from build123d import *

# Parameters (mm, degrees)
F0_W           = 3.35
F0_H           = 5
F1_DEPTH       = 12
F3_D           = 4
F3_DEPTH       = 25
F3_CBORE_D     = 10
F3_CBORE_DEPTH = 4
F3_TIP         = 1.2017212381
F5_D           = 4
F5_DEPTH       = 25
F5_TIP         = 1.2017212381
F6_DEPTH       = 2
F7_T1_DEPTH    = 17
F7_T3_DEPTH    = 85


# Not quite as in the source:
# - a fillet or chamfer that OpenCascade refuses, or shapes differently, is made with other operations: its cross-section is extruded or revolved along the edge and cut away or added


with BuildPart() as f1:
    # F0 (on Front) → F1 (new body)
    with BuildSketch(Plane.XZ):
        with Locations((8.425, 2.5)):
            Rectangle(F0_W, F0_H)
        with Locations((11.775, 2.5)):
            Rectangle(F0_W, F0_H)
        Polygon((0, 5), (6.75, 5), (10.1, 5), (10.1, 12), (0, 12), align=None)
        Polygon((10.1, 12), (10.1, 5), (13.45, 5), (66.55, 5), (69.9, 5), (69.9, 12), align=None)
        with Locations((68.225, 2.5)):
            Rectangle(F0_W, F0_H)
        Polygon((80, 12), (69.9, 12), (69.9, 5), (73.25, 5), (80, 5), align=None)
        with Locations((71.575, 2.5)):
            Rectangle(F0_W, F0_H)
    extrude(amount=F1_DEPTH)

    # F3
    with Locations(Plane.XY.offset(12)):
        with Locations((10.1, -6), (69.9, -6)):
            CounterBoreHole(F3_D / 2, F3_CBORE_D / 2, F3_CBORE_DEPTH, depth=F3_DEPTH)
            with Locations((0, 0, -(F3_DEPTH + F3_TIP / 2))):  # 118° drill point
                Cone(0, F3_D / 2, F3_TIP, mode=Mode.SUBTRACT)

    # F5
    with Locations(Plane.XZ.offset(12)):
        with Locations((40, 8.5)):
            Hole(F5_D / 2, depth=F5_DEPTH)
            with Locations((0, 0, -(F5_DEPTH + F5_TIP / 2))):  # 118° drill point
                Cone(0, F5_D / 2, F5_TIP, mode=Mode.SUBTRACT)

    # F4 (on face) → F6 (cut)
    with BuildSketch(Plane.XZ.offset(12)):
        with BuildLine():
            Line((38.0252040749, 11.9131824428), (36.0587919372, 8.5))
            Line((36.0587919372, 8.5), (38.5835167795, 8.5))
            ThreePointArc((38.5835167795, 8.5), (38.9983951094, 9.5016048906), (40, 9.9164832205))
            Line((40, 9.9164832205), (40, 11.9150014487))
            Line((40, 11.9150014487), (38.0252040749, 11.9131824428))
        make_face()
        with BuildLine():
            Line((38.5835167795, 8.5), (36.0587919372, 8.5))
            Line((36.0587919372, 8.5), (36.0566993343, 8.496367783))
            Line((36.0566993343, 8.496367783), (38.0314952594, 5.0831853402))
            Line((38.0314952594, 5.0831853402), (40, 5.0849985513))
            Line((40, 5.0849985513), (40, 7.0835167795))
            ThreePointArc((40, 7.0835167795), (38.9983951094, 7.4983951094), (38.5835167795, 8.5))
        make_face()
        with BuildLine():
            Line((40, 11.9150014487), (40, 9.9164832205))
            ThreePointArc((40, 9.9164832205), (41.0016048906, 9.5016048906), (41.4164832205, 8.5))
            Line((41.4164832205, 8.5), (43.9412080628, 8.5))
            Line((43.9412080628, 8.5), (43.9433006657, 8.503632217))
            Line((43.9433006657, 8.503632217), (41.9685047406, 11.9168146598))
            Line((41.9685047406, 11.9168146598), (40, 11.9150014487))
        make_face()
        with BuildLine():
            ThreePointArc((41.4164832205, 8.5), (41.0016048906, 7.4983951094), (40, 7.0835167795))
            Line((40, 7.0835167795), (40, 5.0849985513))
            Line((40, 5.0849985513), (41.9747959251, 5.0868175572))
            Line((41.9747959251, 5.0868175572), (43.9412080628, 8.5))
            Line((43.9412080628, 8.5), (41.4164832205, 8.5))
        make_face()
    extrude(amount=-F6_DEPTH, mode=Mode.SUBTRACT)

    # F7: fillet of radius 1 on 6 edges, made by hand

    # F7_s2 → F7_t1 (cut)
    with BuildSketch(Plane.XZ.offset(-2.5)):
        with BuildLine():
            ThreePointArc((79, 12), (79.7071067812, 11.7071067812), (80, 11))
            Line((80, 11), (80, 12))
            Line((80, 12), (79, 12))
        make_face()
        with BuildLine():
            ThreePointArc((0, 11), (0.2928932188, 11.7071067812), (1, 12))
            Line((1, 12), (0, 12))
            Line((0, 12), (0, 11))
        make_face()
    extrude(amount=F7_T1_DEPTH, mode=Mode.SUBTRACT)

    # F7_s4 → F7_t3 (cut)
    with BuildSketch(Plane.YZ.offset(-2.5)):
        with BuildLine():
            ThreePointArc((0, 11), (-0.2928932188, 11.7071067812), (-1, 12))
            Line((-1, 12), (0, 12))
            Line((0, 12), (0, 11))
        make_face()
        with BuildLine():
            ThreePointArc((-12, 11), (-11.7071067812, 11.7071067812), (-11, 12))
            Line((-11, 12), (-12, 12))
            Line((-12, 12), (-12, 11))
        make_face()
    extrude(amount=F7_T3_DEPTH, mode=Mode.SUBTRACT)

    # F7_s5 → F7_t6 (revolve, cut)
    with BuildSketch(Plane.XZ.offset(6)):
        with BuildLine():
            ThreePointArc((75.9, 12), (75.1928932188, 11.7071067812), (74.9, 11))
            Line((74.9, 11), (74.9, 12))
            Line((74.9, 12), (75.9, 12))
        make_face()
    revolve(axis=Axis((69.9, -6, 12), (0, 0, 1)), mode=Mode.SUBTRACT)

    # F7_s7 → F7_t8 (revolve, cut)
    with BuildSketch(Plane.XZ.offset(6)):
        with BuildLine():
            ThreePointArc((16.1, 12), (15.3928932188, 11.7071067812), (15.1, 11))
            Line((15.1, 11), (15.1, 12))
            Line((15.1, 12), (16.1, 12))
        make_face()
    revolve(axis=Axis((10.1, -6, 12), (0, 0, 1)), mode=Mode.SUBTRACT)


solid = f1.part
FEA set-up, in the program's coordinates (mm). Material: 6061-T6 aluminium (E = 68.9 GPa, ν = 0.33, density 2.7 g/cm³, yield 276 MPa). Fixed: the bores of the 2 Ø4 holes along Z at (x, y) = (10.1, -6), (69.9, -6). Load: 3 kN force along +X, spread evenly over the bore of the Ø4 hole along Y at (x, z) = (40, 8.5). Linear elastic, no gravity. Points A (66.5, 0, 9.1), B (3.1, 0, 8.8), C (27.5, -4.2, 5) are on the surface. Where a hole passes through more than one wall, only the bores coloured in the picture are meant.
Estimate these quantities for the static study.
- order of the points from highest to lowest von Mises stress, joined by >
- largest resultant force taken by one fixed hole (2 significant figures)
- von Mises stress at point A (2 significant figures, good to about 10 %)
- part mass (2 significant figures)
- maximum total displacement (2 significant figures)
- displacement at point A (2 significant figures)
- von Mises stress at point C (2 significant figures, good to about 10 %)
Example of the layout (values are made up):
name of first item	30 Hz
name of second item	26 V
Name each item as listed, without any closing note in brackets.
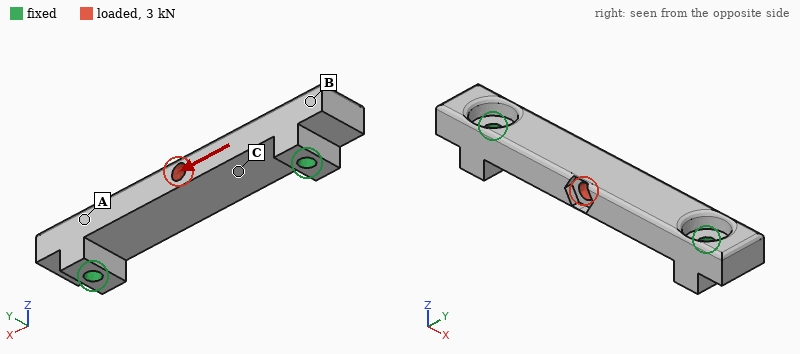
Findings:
order of the points from highest to lowest von Mises stress, joined by >	C > A > B
largest resultant force taken by one fixed hole	1.5 kN
von Mises stress at point A	18 MPa
part mass	17 g
maximum total displacement	12 µm
displacement at point A	4.1 µm
von Mises stress at point C	30 MPa
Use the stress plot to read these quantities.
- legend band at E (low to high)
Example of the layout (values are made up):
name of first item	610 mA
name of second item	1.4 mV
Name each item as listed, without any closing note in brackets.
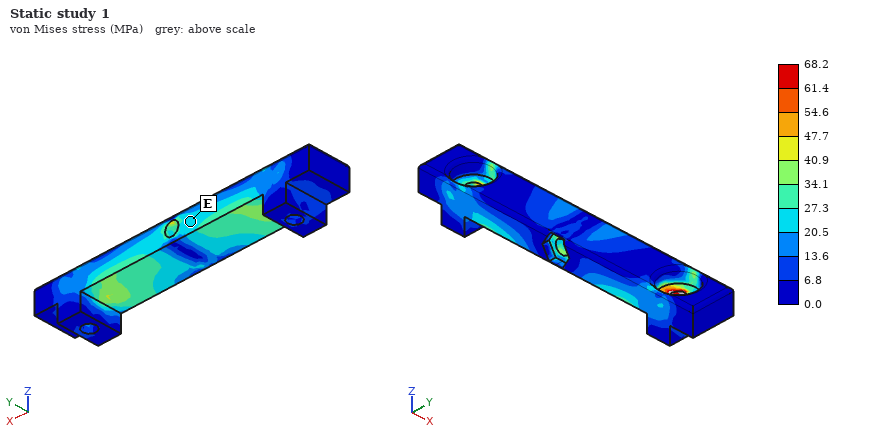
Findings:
legend band at E	20.5 to 27.3 MPa
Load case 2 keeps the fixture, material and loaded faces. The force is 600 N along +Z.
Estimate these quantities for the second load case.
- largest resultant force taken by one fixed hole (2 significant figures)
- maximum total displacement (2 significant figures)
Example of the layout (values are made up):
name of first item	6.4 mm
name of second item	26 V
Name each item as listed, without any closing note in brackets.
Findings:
largest resultant force taken by one fixed hole	540 N
maximum total displacement	48 µm
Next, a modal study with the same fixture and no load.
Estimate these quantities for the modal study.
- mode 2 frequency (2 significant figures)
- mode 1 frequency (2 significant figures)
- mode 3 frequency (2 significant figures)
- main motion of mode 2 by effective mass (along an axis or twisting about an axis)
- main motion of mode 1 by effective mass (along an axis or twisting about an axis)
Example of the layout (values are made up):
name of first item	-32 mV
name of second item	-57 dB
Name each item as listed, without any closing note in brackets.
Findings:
mode 2 frequency	10 kHz
mode 1 frequency	8300 Hz
mode 3 frequency	19 kHz
main motion of mode 2 by effective mass	along Y
main motion of mode 1 by effective mass	along Z
